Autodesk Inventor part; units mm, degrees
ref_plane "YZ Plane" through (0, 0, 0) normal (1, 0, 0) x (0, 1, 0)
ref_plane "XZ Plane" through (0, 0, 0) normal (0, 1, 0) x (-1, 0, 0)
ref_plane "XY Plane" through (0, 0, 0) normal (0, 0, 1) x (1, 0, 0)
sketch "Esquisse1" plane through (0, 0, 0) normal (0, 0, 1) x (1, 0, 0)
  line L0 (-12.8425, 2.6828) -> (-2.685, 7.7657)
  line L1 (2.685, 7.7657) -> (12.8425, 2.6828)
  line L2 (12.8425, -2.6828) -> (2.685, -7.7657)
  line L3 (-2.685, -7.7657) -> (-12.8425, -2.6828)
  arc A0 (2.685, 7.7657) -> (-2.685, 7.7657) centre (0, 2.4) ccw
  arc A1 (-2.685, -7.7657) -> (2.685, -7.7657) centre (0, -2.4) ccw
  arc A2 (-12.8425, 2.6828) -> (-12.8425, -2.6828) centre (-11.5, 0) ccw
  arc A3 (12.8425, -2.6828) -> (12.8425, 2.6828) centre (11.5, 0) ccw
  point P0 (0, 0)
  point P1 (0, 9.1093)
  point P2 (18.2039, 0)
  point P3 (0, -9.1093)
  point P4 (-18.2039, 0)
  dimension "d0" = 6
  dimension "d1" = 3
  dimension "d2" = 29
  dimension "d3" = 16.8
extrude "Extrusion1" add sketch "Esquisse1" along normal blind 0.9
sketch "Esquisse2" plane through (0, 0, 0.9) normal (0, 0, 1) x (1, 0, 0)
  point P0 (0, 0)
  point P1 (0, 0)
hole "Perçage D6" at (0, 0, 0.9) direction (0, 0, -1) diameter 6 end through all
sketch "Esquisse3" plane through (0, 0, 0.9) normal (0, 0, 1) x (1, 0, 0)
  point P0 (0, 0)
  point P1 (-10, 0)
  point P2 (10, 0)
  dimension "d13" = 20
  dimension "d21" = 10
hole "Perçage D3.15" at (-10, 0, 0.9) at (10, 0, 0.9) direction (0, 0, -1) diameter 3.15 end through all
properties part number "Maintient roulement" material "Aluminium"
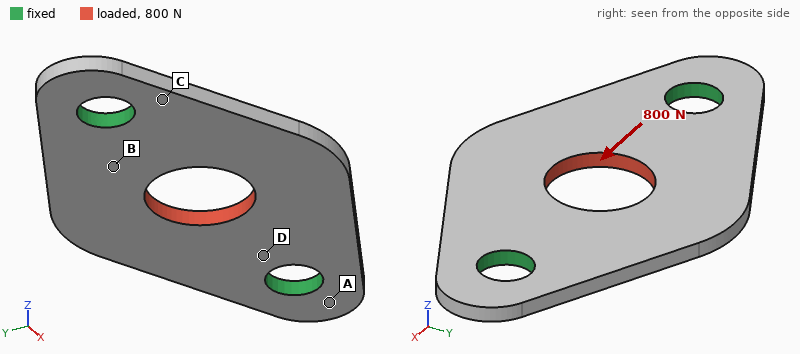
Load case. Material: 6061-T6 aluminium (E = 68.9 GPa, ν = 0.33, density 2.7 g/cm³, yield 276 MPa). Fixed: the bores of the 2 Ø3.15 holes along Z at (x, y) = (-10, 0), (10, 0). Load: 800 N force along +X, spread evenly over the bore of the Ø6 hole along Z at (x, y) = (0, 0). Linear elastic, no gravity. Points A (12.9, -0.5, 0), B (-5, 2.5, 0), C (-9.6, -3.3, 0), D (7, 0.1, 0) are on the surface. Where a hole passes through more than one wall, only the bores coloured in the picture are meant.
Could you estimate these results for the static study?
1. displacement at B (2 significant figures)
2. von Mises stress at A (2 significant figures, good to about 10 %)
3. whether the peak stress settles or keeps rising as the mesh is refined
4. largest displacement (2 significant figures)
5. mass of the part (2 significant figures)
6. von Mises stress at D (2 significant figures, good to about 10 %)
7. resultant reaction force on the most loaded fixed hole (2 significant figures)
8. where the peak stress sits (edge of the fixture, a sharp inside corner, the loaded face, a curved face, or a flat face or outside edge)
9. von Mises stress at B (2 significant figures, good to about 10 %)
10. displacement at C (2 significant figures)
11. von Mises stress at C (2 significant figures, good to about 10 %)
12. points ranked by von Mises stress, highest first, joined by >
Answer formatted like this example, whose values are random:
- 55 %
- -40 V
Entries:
- 4.2 µm
- 14 MPa
- keeps rising
- 7.4 µm
- 0.65 g
- 78 MPa
- 400 N
- edge of the fixture
- 54 MPa
- 2.0 µm
- 29 MPa
- D > B > C > A
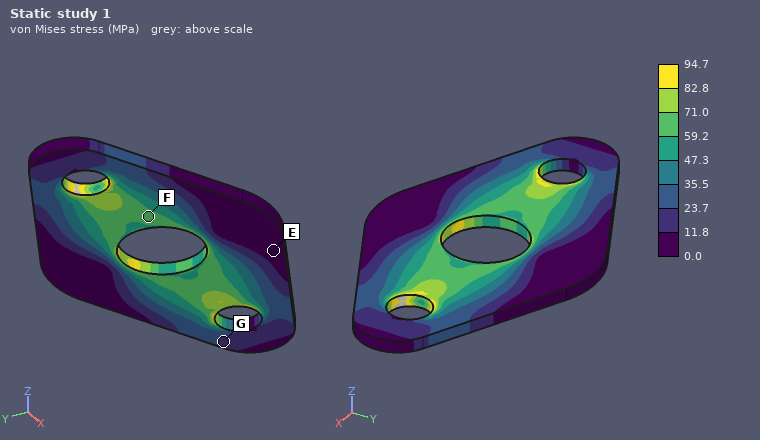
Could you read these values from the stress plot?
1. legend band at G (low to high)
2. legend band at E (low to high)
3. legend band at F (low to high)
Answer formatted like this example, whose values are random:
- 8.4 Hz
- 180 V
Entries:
- 11.8 to 23.7 MPa
- 0.0 to 11.8 MPa
- 59.2 to 71.0 MPa
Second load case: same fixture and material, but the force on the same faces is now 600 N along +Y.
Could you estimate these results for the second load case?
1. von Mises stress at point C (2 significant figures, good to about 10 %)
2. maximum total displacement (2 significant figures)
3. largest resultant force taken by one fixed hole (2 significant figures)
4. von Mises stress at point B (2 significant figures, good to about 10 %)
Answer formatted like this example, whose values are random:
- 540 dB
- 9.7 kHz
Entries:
- 20 MPa
- 12 µm
- 300 N
- 47 MPa
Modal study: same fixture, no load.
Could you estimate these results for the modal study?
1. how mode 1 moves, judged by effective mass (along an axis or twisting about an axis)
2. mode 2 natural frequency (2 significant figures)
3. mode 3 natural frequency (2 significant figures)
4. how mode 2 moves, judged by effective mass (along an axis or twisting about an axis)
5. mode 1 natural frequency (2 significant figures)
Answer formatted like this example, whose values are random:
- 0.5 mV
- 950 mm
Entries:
- twisting about X
- 10 kHz
- 27 kHz
- along Z
- 9600 Hz
